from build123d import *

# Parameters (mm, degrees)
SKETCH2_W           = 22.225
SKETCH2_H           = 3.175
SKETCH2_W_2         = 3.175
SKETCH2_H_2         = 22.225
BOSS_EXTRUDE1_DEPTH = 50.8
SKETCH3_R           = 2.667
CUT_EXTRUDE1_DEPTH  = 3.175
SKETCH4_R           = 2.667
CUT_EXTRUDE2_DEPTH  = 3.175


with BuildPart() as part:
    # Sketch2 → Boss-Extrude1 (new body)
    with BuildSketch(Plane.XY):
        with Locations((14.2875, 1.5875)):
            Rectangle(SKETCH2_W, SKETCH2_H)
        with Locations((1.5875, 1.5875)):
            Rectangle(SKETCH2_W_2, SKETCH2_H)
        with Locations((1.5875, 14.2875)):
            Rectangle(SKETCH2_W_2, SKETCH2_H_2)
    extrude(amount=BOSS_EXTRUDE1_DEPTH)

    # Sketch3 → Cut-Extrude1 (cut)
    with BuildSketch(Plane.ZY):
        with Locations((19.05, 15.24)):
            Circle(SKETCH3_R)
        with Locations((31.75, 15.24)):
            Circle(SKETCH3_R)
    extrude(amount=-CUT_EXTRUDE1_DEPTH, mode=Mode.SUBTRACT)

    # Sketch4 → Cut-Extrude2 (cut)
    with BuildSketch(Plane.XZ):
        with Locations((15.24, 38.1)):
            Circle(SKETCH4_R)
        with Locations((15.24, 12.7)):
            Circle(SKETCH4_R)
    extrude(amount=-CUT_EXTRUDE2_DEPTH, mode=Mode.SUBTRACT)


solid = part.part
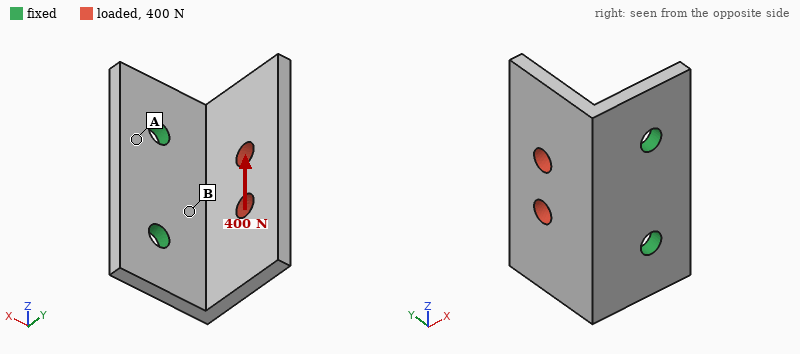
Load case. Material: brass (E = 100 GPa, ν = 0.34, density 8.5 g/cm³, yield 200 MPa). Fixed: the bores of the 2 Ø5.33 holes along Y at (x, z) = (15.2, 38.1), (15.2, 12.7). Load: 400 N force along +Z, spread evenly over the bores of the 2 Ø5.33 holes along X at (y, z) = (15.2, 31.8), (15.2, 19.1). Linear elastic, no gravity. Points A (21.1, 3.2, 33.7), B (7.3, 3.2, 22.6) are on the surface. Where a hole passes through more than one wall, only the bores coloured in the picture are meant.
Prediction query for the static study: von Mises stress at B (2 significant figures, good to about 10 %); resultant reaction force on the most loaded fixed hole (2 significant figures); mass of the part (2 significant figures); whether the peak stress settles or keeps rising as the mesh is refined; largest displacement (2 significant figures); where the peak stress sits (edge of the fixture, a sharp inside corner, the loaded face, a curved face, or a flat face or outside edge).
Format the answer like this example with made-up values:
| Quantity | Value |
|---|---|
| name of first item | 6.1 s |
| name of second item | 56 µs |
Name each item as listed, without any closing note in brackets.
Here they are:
| Quantity | Value |
|---|---|
| von Mises stress at B | 22 MPa |
| resultant reaction force on the most loaded fixed hole | 320 N |
| mass of the part | 63 g |
| whether the peak stress settles or keeps rising as the mesh is refined | keeps rising |
| largest displacement | 37 µm |
| where the peak stress sits | edge of the fixture |
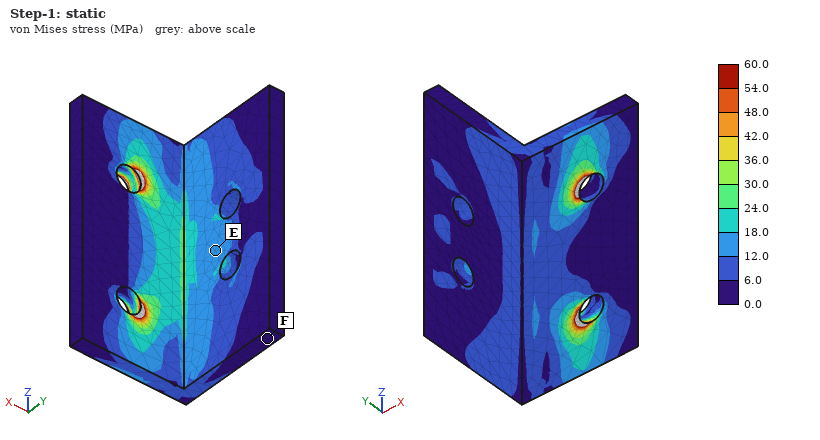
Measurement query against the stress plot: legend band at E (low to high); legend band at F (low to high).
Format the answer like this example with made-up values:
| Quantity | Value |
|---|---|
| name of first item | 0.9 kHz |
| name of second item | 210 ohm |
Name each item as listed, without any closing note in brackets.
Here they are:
| Quantity | Value |
|---|---|
| legend band at E | 12.0 to 18.0 MPa |
| legend band at F | 0.0 to 6.0 MPa |
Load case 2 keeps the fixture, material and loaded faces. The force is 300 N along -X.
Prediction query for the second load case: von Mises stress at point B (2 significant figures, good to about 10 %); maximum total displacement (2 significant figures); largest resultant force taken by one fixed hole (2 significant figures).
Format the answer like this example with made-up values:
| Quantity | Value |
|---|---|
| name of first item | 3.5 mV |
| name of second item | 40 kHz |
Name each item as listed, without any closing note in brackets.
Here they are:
| Quantity | Value |
|---|---|
| von Mises stress at point B | 47 MPa |
| maximum total displacement | 0.13 mm |
| largest resultant force taken by one fixed hole | 160 N |
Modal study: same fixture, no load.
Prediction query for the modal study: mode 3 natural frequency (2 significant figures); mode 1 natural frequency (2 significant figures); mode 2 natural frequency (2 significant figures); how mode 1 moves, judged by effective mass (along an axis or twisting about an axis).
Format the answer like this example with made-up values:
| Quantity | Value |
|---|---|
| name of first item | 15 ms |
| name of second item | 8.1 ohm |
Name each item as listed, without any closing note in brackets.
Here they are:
| Quantity | Value |
|---|---|
| mode 3 natural frequency | 4600 Hz |
| mode 1 natural frequency | 1700 Hz |
| mode 2 natural frequency | 2800 Hz |
| how mode 1 moves, judged by effective mass | along X |
